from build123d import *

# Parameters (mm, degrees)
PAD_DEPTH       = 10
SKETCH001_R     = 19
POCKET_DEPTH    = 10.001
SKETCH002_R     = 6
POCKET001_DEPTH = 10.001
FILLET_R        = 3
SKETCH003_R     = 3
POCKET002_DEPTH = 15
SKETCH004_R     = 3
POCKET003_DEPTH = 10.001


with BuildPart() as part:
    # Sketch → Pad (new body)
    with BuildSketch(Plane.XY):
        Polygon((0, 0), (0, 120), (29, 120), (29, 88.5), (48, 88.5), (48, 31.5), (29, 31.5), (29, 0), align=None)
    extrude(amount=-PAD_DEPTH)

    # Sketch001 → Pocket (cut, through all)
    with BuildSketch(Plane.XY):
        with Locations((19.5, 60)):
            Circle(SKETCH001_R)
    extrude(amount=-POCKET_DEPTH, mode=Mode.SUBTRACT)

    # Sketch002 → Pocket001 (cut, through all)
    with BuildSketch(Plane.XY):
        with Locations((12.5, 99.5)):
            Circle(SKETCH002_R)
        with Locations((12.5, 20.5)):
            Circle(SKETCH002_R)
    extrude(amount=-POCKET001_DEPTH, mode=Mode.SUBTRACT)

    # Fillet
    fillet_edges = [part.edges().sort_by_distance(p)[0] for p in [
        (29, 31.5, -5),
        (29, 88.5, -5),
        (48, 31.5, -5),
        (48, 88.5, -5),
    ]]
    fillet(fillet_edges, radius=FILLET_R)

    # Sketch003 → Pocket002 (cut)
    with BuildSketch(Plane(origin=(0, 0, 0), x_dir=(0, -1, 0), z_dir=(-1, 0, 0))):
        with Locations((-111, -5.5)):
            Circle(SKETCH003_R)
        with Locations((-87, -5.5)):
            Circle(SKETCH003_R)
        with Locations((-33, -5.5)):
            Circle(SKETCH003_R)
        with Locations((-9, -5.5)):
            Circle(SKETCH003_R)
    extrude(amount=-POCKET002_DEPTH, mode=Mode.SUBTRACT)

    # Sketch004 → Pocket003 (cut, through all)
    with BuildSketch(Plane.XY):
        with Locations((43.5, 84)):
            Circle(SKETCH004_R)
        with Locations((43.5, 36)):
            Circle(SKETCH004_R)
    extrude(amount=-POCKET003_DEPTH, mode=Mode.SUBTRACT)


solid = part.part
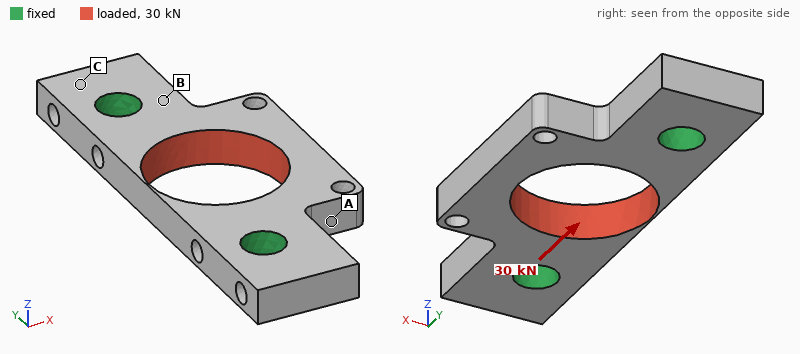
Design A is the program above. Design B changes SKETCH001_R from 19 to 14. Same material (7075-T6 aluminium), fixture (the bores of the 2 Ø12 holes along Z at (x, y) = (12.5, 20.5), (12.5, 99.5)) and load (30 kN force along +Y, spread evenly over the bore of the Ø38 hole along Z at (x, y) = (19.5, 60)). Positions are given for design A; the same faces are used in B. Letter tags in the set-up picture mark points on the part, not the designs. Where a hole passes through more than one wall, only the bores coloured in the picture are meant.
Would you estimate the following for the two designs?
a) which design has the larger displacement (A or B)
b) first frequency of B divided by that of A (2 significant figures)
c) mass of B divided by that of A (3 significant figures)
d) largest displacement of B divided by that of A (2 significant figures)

A
1.00
1.17
0.62
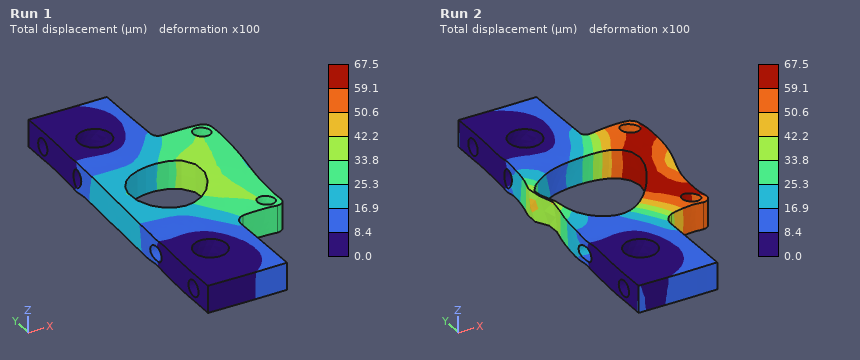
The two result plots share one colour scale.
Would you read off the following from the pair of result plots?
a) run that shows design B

Run 1
